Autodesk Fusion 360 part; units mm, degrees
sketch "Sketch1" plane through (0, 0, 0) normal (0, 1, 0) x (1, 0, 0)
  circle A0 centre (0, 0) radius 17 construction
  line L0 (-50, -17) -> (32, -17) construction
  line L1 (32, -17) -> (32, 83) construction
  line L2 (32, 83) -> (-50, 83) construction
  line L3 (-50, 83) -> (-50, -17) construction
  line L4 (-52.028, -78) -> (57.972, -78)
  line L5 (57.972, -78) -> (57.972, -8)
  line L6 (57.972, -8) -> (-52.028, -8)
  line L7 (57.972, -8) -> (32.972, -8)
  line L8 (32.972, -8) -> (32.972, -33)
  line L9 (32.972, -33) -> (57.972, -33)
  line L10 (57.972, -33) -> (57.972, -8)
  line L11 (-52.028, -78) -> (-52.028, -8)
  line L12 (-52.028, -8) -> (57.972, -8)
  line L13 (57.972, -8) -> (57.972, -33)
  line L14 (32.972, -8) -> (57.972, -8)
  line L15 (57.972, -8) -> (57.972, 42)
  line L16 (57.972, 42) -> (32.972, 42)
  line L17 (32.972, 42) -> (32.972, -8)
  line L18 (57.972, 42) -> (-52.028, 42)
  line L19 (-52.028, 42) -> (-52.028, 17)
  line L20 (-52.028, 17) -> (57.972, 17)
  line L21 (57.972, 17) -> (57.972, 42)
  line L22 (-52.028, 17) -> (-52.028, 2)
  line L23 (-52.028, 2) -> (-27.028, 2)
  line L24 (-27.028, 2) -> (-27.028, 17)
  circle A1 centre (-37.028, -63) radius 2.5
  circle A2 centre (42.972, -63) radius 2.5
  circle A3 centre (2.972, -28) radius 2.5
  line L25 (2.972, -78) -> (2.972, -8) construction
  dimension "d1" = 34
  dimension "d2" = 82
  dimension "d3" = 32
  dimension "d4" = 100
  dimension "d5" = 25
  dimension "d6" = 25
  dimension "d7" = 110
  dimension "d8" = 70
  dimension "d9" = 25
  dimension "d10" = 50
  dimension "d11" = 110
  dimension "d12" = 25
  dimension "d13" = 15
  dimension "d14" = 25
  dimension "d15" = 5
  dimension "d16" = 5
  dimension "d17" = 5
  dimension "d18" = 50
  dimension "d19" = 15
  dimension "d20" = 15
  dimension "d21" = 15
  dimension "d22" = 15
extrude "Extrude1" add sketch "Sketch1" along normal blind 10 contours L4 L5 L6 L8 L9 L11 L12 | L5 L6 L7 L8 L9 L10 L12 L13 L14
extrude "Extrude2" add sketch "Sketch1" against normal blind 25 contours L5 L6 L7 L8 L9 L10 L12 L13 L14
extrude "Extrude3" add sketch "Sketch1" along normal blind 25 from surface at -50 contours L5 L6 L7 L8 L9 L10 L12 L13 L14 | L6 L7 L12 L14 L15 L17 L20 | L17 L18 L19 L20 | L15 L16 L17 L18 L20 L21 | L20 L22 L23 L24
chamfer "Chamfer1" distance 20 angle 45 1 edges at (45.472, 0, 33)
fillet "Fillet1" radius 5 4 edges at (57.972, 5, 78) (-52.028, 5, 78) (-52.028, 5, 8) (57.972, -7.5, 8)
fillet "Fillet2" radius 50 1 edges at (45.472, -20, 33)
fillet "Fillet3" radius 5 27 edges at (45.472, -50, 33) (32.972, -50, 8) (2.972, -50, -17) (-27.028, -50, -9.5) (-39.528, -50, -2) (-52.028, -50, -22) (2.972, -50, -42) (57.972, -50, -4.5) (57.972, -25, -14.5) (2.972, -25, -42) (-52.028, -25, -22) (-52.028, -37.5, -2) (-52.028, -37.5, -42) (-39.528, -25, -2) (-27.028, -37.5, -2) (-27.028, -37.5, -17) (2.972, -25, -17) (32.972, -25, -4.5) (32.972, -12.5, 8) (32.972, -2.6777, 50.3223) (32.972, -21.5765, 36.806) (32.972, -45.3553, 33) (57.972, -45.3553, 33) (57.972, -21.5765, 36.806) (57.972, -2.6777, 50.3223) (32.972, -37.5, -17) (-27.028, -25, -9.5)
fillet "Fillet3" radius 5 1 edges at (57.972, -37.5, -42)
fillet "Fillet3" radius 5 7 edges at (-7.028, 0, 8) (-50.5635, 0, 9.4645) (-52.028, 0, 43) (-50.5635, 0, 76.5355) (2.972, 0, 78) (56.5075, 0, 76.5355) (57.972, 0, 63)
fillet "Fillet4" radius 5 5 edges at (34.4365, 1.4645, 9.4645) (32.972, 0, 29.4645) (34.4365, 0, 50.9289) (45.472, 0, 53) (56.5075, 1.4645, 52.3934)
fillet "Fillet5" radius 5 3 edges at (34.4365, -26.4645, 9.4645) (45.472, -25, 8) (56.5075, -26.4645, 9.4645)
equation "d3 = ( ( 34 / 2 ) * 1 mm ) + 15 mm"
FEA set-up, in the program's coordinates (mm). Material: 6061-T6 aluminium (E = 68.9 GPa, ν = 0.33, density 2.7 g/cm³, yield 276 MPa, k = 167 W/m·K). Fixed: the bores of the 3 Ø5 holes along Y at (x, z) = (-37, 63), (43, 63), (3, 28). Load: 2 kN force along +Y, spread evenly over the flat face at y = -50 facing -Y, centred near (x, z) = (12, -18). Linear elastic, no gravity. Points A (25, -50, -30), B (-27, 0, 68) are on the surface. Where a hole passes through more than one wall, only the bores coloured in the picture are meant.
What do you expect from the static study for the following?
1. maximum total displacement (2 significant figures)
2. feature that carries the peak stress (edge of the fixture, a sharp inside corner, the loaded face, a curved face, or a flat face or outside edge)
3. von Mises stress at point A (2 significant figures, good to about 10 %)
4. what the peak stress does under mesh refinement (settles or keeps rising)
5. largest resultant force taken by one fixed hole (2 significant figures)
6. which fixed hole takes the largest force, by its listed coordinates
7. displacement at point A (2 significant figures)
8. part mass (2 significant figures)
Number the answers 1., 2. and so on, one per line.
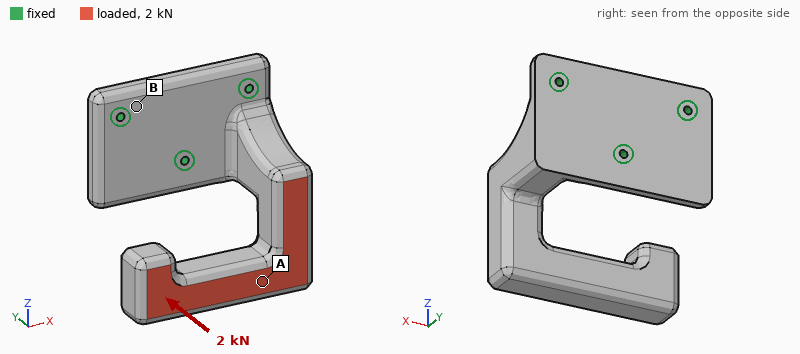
1. 0.67 mm
2. edge of the fixture
3. 17 MPa
4. keeps rising
5. 3.5 kN
6. (3, 28)
7. 0.43 mm
8. 540 g
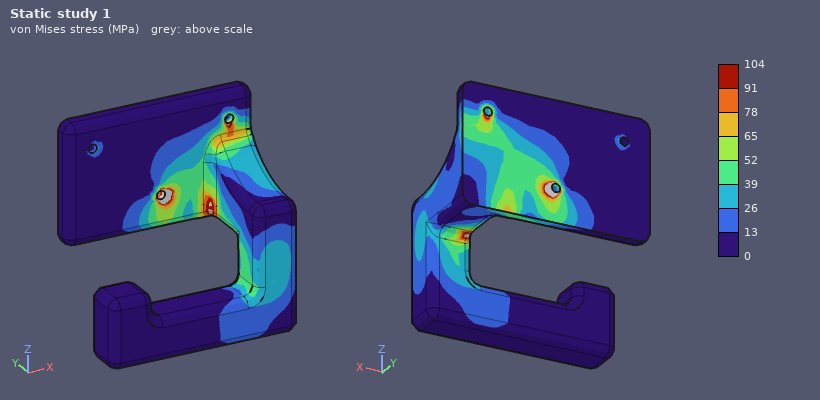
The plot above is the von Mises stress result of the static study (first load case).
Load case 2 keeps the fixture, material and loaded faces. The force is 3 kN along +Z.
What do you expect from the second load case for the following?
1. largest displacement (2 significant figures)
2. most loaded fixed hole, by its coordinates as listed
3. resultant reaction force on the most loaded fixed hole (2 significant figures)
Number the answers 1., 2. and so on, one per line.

1. 0.94 mm
2. (3, 28)
3. 3.3 kN
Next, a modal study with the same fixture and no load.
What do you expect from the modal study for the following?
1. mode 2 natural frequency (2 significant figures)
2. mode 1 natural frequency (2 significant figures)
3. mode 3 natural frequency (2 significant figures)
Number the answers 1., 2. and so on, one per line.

1. 650 Hz
2. 560 Hz
3. 1100 Hz
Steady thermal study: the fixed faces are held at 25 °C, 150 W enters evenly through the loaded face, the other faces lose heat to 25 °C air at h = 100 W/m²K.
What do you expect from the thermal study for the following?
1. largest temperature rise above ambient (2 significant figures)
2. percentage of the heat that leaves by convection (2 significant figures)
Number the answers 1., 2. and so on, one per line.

1. 73 K
2. 62 %
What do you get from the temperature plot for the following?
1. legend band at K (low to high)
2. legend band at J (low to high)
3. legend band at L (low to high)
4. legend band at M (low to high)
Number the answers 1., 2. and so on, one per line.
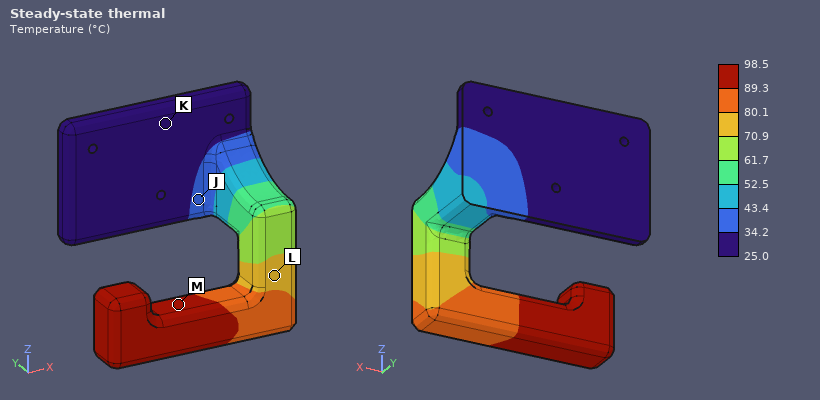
1. 25.0 to 34.2 °C
2. 34.2 to 43.4 °C
3. 70.9 to 80.1 °C
4. 89.3 to 98.5 °C
